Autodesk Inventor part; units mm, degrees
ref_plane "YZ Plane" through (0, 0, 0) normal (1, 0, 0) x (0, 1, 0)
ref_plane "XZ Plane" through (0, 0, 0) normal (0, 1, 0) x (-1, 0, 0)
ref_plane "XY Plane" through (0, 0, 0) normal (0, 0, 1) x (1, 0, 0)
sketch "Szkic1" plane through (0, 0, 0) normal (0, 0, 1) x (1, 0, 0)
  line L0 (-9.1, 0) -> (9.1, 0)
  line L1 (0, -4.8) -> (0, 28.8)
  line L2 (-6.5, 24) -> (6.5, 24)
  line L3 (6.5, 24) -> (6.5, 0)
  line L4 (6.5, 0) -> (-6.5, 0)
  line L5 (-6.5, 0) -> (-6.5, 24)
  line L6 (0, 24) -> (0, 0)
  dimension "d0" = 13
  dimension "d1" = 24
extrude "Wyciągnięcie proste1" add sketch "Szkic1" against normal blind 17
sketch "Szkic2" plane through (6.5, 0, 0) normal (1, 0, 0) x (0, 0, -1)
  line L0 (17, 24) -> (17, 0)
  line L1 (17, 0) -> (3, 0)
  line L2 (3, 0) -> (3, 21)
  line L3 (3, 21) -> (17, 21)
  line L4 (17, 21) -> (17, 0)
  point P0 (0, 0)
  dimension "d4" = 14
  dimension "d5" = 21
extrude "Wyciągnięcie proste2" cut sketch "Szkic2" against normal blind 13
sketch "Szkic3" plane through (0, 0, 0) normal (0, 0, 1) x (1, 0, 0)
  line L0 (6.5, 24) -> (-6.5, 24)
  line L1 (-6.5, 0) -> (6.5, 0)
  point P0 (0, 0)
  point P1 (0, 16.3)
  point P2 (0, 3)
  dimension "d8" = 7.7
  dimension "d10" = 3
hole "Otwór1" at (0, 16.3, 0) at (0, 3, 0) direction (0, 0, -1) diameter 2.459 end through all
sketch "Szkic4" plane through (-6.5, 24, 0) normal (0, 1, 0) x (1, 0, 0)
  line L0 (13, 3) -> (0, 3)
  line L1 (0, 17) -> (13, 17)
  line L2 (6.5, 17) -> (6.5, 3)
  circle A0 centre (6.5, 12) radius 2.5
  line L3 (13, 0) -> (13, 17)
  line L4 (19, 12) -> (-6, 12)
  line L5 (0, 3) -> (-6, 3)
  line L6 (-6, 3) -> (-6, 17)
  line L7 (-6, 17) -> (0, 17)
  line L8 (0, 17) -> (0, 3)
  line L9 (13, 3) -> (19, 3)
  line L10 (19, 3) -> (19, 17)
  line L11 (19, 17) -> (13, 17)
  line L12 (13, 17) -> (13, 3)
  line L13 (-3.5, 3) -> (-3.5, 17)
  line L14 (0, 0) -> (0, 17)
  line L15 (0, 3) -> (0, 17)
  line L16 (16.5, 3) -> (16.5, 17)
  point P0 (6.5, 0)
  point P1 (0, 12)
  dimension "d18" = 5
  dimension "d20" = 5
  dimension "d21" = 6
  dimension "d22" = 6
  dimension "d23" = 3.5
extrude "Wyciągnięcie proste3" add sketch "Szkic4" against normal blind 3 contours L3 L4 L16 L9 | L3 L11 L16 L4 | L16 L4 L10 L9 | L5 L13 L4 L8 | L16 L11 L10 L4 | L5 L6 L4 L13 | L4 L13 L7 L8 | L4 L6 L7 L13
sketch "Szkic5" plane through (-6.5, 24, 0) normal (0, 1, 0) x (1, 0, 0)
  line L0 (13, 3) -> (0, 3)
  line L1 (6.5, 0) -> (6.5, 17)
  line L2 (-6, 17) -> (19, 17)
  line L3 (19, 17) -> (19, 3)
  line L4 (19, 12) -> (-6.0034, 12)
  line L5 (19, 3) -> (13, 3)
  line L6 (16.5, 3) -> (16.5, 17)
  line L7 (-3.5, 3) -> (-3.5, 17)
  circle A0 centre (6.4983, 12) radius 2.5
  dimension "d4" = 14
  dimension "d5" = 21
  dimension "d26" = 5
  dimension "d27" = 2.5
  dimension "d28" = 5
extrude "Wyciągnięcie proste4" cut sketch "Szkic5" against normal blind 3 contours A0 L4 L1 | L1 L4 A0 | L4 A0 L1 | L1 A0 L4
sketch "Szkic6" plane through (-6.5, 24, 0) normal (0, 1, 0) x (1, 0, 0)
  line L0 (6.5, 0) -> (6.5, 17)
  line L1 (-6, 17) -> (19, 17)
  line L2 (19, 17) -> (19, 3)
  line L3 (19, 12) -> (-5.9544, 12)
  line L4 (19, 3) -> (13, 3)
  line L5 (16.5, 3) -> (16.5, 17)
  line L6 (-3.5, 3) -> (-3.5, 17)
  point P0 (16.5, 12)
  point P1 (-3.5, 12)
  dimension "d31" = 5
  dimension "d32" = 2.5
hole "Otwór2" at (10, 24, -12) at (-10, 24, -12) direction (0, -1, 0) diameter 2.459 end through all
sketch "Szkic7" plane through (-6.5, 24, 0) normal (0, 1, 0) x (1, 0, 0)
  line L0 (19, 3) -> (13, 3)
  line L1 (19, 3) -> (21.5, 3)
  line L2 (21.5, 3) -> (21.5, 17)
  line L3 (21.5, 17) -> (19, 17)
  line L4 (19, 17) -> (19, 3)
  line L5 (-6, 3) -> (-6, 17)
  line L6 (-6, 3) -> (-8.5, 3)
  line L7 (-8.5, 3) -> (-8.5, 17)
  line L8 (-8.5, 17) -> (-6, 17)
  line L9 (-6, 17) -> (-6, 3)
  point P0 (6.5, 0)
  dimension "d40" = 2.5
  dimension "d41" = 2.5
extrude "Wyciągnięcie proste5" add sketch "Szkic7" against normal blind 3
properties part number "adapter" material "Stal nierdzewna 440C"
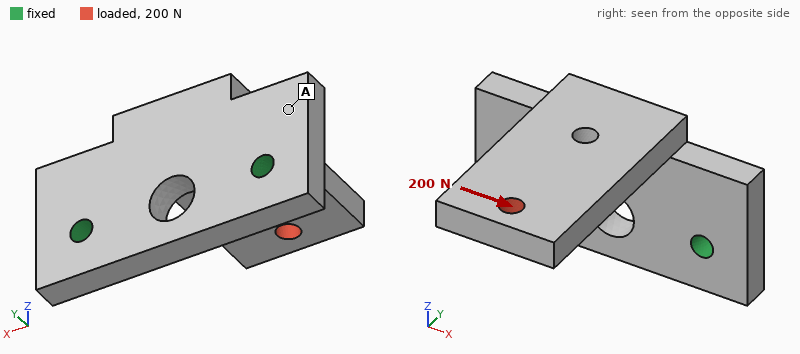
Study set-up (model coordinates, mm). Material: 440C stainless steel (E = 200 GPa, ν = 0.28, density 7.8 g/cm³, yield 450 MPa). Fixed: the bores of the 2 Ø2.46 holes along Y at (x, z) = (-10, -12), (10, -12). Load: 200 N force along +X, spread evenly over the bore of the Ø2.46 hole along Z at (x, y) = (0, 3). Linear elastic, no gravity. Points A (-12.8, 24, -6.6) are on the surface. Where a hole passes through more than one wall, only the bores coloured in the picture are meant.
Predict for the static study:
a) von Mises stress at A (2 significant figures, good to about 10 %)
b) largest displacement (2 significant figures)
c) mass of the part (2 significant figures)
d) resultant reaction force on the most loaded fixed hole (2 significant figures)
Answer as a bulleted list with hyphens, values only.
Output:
- 24 MPa
- 43 µm
- 16 g
- 260 N
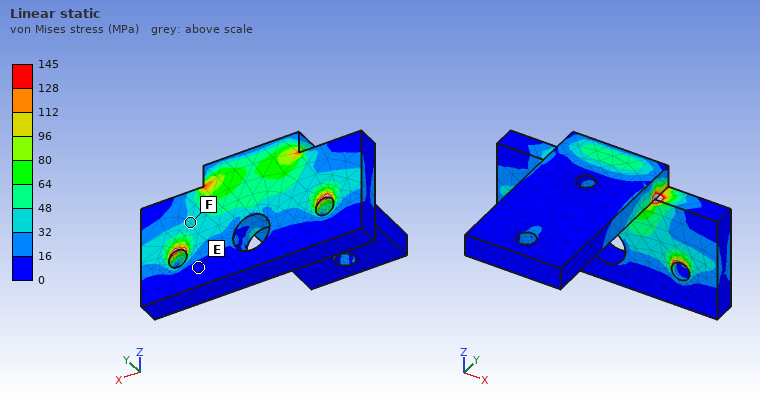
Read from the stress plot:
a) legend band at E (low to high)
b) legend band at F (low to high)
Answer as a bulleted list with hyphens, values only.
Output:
- 0 to 16 MPa
- 32 to 48 MPa
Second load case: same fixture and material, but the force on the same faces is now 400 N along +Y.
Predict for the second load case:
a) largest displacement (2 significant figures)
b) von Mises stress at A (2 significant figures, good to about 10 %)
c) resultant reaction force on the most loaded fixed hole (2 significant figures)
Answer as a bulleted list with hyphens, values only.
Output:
- 67 µm
- 51 MPa
- 200 N
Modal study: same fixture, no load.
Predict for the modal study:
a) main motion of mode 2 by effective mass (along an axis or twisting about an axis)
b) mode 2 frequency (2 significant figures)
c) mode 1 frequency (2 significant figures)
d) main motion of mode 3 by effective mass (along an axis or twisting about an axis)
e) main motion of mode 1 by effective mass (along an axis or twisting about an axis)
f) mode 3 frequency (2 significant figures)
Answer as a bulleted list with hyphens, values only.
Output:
- along X
- 6800 Hz
- 3100 Hz
- along Y
- along Z
- 9900 Hz
